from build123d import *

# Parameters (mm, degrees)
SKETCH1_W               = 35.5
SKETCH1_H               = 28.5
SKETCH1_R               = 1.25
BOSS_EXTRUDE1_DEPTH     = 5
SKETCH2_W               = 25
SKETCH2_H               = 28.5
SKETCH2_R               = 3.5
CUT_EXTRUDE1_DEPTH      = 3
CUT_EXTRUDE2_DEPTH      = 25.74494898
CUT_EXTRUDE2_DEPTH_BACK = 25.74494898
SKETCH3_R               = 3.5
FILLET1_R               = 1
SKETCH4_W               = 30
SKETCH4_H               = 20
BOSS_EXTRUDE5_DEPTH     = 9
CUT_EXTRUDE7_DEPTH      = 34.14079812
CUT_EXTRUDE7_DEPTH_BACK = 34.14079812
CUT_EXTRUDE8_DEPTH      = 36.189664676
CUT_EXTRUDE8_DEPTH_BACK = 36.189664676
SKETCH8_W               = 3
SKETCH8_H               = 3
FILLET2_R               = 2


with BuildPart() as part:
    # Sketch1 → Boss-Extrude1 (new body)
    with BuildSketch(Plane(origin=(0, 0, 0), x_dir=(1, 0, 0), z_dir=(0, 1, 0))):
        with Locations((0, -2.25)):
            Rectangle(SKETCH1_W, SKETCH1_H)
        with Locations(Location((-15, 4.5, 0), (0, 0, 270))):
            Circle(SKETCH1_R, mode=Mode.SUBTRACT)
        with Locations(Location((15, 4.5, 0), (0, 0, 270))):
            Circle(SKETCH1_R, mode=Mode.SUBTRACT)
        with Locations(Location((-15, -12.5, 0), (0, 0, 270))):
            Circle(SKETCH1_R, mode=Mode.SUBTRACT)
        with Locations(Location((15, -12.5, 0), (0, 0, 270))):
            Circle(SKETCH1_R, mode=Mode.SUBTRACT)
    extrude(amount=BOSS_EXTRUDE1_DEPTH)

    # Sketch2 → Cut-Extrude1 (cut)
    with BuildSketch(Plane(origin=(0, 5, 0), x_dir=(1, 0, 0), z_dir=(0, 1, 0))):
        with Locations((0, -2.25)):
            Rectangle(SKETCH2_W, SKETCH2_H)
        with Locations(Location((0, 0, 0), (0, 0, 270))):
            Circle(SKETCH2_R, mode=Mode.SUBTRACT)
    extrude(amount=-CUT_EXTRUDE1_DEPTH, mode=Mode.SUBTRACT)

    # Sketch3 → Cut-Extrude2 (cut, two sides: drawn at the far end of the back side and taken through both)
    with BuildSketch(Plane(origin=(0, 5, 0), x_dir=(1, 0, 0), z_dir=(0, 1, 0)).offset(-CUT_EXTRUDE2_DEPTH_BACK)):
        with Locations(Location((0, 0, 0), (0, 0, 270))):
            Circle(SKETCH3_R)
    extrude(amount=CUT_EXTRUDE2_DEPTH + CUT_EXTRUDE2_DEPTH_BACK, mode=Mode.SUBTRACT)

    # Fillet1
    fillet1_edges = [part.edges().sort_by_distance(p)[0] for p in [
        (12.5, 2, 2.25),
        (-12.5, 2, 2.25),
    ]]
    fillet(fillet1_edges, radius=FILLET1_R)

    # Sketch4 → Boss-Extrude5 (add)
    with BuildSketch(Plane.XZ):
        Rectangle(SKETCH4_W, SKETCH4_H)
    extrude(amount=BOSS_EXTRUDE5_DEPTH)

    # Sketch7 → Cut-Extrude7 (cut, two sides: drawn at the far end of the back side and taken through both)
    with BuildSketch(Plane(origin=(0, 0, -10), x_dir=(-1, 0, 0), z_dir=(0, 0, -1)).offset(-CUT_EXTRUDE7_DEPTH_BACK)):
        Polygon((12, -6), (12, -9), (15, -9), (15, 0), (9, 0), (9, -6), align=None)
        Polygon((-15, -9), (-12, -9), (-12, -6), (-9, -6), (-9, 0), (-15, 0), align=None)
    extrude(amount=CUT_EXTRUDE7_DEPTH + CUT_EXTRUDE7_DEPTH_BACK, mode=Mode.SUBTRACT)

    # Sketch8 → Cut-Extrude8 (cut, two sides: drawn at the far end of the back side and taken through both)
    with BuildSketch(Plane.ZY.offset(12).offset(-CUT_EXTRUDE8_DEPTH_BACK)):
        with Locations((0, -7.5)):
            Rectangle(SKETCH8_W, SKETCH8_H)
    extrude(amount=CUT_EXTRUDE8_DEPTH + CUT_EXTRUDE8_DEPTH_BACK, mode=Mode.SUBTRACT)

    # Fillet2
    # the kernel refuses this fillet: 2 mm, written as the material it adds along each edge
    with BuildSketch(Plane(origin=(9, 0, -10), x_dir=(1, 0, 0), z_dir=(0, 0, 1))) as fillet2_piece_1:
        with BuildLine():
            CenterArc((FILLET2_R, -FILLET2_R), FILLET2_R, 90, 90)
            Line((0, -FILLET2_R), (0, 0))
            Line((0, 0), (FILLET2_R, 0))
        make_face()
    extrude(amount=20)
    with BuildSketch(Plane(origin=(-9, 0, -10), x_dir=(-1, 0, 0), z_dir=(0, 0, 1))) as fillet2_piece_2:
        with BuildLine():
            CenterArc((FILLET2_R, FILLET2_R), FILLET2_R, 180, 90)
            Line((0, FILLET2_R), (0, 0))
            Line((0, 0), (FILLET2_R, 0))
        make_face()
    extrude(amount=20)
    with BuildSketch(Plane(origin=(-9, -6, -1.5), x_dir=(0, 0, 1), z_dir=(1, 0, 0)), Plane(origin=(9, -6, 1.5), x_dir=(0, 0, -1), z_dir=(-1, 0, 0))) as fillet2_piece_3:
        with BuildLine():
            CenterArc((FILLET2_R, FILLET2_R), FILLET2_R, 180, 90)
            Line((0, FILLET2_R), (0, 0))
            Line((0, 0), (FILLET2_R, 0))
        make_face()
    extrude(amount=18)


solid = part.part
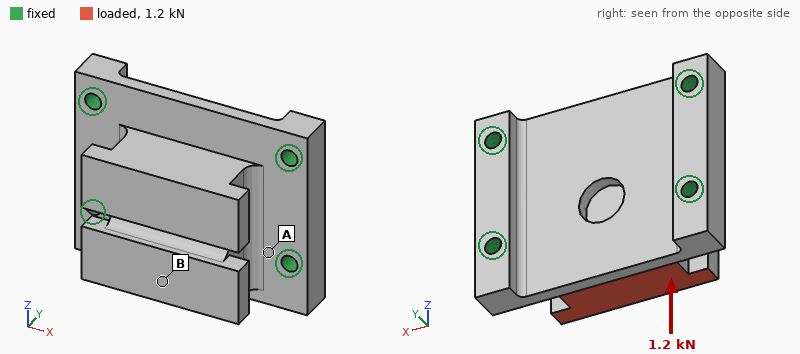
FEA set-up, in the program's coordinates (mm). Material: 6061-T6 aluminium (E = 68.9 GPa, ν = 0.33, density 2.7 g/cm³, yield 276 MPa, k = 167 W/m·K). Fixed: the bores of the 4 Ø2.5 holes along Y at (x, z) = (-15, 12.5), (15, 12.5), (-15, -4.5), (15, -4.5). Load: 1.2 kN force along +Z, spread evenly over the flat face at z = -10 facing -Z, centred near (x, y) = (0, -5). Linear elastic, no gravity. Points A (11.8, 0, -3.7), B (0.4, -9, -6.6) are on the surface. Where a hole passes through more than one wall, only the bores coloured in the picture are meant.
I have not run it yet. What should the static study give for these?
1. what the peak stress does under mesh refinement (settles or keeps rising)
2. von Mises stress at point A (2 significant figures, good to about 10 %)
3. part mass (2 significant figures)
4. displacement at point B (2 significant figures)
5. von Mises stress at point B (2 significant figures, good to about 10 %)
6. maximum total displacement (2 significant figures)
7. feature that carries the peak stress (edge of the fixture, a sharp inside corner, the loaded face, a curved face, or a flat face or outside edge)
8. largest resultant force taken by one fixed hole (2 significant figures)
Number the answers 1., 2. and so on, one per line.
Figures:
1. keeps rising
2. 35 MPa
3. 17 g
4. 16 µm
5. 8.9 MPa
6. 19 µm
7. a sharp inside corner
8. 460 N
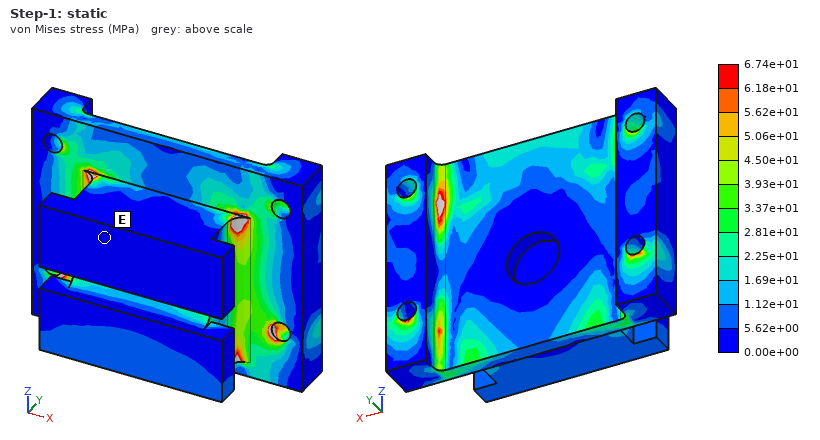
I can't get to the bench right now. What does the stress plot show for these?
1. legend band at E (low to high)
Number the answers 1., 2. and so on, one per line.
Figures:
1. 0.00e+00 to 5.62e+00 MPa
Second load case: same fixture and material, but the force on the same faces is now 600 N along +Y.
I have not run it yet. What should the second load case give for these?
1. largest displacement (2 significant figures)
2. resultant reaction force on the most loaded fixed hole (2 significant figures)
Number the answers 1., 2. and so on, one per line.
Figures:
1. 18 µm
2. 470 N
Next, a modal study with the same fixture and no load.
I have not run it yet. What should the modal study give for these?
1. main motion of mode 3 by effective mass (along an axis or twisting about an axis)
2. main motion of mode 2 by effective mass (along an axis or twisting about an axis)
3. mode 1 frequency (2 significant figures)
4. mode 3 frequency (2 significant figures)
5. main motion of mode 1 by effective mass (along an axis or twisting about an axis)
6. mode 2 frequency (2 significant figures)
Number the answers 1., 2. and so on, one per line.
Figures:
1. along X
2. along Y
3. 14 kHz
4. 24 kHz
5. along Z
6. 17 kHz
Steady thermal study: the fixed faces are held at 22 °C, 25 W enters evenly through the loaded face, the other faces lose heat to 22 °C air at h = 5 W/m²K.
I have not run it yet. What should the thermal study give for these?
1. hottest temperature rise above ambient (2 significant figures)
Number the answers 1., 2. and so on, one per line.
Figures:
1. 18 K
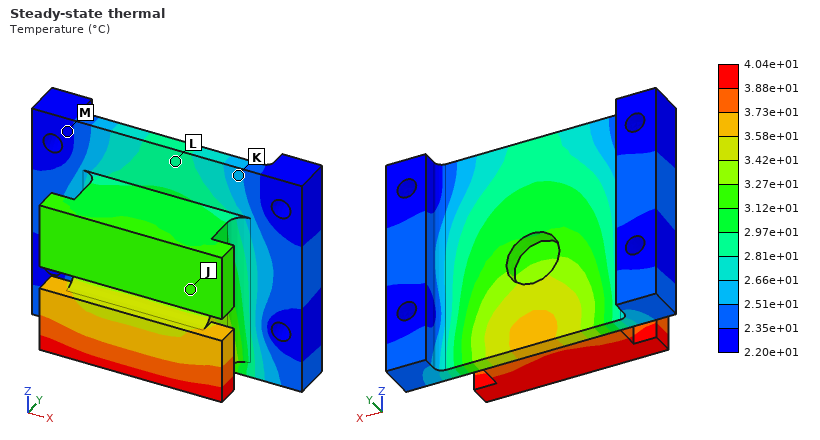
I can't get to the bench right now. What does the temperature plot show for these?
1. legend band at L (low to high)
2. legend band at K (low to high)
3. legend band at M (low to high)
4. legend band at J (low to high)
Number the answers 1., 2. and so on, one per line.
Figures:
1. 2.81e+01 to 2.97e+01 °C
2. 2.51e+01 to 2.66e+01 °C
3. 2.20e+01 to 2.35e+01 °C
4. 3.12e+01 to 3.27e+01 °C
